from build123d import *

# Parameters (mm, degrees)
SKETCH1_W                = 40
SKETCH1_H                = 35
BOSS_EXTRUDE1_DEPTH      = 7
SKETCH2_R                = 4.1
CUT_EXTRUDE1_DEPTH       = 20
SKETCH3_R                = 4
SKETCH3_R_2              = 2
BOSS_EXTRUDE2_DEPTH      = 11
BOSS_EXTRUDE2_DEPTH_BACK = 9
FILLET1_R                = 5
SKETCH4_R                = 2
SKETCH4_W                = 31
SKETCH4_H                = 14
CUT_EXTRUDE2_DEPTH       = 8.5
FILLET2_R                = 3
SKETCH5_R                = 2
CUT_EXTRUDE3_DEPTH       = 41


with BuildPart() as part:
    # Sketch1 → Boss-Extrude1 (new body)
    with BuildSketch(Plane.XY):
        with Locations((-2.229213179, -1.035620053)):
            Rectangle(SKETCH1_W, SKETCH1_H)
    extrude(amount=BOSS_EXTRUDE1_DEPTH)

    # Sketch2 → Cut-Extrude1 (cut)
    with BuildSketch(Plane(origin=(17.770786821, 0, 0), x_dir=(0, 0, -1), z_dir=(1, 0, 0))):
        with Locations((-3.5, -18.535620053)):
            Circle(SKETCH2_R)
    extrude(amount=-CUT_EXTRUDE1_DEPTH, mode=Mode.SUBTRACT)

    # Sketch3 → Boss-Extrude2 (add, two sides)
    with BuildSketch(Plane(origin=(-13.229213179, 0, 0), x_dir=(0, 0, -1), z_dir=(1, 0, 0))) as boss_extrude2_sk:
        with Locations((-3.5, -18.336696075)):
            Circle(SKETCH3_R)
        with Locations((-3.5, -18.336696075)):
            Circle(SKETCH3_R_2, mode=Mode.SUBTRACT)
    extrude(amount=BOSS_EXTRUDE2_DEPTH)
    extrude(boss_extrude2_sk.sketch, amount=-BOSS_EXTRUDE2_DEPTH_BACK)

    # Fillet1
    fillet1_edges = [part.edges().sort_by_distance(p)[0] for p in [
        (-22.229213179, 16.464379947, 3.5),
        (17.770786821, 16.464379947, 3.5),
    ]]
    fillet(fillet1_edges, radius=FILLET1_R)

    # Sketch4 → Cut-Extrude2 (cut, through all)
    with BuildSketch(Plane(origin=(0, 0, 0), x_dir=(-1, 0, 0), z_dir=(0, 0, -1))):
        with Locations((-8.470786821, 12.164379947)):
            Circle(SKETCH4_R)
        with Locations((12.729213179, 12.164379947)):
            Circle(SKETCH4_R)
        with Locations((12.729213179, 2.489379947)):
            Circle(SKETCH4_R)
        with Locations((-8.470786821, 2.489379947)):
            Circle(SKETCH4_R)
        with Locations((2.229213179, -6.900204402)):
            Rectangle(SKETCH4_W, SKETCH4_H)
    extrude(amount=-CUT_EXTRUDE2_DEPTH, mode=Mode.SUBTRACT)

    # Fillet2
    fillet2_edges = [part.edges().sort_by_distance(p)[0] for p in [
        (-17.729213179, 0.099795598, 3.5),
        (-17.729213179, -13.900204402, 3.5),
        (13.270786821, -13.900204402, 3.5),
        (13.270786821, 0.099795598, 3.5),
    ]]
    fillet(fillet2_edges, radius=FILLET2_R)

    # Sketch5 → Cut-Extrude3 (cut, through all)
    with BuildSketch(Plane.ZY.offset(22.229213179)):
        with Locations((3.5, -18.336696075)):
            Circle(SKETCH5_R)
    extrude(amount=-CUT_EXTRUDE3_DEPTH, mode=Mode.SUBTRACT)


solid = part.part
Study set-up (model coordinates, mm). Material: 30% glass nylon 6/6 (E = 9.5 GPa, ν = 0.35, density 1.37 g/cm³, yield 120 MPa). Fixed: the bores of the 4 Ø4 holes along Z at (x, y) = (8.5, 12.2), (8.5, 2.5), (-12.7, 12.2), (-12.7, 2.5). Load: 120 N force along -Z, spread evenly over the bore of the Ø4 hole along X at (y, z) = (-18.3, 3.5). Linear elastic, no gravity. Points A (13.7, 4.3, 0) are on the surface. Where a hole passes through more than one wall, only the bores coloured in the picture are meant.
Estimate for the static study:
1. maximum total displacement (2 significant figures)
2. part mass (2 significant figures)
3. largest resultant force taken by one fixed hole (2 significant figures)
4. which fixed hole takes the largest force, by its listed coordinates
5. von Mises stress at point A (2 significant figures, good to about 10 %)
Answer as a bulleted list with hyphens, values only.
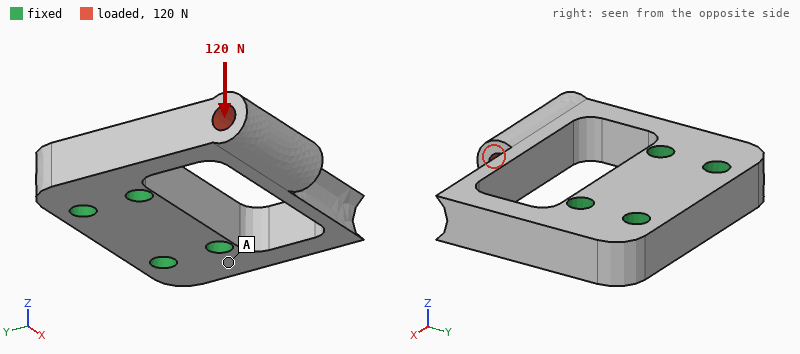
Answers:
- 0.41 mm
- 8.4 g
- 190 N
- (-12.7, 2.5)
- 5.8 MPa
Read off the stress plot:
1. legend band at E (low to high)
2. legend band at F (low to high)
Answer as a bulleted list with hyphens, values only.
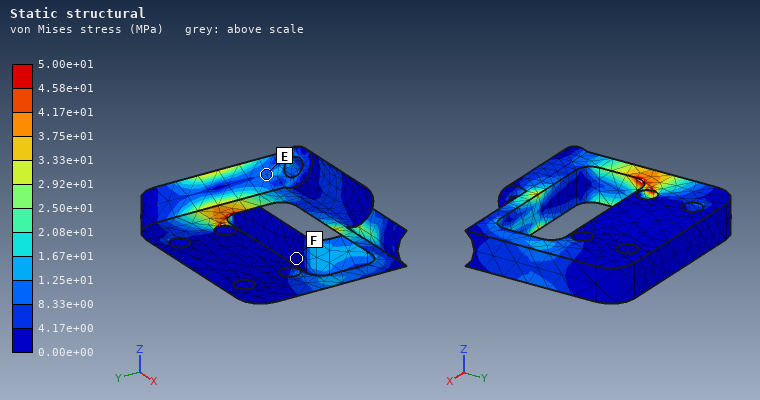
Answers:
- 8.33e+00 to 1.25e+01 MPa
- 0.00e+00 to 4.17e+00 MPa
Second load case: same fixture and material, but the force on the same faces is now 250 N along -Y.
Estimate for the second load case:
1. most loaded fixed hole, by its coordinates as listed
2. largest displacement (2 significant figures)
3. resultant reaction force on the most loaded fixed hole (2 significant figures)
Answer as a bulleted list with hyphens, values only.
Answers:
- (-12.7, 2.5)
- 0.42 mm
- 190 N
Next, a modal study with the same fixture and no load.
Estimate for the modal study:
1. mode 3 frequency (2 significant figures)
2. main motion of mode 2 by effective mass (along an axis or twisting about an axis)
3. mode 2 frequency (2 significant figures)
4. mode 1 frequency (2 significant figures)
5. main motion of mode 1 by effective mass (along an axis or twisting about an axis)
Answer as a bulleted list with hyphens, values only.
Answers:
- 5700 Hz
- along X
- 3000 Hz
- 2700 Hz
- along Z
